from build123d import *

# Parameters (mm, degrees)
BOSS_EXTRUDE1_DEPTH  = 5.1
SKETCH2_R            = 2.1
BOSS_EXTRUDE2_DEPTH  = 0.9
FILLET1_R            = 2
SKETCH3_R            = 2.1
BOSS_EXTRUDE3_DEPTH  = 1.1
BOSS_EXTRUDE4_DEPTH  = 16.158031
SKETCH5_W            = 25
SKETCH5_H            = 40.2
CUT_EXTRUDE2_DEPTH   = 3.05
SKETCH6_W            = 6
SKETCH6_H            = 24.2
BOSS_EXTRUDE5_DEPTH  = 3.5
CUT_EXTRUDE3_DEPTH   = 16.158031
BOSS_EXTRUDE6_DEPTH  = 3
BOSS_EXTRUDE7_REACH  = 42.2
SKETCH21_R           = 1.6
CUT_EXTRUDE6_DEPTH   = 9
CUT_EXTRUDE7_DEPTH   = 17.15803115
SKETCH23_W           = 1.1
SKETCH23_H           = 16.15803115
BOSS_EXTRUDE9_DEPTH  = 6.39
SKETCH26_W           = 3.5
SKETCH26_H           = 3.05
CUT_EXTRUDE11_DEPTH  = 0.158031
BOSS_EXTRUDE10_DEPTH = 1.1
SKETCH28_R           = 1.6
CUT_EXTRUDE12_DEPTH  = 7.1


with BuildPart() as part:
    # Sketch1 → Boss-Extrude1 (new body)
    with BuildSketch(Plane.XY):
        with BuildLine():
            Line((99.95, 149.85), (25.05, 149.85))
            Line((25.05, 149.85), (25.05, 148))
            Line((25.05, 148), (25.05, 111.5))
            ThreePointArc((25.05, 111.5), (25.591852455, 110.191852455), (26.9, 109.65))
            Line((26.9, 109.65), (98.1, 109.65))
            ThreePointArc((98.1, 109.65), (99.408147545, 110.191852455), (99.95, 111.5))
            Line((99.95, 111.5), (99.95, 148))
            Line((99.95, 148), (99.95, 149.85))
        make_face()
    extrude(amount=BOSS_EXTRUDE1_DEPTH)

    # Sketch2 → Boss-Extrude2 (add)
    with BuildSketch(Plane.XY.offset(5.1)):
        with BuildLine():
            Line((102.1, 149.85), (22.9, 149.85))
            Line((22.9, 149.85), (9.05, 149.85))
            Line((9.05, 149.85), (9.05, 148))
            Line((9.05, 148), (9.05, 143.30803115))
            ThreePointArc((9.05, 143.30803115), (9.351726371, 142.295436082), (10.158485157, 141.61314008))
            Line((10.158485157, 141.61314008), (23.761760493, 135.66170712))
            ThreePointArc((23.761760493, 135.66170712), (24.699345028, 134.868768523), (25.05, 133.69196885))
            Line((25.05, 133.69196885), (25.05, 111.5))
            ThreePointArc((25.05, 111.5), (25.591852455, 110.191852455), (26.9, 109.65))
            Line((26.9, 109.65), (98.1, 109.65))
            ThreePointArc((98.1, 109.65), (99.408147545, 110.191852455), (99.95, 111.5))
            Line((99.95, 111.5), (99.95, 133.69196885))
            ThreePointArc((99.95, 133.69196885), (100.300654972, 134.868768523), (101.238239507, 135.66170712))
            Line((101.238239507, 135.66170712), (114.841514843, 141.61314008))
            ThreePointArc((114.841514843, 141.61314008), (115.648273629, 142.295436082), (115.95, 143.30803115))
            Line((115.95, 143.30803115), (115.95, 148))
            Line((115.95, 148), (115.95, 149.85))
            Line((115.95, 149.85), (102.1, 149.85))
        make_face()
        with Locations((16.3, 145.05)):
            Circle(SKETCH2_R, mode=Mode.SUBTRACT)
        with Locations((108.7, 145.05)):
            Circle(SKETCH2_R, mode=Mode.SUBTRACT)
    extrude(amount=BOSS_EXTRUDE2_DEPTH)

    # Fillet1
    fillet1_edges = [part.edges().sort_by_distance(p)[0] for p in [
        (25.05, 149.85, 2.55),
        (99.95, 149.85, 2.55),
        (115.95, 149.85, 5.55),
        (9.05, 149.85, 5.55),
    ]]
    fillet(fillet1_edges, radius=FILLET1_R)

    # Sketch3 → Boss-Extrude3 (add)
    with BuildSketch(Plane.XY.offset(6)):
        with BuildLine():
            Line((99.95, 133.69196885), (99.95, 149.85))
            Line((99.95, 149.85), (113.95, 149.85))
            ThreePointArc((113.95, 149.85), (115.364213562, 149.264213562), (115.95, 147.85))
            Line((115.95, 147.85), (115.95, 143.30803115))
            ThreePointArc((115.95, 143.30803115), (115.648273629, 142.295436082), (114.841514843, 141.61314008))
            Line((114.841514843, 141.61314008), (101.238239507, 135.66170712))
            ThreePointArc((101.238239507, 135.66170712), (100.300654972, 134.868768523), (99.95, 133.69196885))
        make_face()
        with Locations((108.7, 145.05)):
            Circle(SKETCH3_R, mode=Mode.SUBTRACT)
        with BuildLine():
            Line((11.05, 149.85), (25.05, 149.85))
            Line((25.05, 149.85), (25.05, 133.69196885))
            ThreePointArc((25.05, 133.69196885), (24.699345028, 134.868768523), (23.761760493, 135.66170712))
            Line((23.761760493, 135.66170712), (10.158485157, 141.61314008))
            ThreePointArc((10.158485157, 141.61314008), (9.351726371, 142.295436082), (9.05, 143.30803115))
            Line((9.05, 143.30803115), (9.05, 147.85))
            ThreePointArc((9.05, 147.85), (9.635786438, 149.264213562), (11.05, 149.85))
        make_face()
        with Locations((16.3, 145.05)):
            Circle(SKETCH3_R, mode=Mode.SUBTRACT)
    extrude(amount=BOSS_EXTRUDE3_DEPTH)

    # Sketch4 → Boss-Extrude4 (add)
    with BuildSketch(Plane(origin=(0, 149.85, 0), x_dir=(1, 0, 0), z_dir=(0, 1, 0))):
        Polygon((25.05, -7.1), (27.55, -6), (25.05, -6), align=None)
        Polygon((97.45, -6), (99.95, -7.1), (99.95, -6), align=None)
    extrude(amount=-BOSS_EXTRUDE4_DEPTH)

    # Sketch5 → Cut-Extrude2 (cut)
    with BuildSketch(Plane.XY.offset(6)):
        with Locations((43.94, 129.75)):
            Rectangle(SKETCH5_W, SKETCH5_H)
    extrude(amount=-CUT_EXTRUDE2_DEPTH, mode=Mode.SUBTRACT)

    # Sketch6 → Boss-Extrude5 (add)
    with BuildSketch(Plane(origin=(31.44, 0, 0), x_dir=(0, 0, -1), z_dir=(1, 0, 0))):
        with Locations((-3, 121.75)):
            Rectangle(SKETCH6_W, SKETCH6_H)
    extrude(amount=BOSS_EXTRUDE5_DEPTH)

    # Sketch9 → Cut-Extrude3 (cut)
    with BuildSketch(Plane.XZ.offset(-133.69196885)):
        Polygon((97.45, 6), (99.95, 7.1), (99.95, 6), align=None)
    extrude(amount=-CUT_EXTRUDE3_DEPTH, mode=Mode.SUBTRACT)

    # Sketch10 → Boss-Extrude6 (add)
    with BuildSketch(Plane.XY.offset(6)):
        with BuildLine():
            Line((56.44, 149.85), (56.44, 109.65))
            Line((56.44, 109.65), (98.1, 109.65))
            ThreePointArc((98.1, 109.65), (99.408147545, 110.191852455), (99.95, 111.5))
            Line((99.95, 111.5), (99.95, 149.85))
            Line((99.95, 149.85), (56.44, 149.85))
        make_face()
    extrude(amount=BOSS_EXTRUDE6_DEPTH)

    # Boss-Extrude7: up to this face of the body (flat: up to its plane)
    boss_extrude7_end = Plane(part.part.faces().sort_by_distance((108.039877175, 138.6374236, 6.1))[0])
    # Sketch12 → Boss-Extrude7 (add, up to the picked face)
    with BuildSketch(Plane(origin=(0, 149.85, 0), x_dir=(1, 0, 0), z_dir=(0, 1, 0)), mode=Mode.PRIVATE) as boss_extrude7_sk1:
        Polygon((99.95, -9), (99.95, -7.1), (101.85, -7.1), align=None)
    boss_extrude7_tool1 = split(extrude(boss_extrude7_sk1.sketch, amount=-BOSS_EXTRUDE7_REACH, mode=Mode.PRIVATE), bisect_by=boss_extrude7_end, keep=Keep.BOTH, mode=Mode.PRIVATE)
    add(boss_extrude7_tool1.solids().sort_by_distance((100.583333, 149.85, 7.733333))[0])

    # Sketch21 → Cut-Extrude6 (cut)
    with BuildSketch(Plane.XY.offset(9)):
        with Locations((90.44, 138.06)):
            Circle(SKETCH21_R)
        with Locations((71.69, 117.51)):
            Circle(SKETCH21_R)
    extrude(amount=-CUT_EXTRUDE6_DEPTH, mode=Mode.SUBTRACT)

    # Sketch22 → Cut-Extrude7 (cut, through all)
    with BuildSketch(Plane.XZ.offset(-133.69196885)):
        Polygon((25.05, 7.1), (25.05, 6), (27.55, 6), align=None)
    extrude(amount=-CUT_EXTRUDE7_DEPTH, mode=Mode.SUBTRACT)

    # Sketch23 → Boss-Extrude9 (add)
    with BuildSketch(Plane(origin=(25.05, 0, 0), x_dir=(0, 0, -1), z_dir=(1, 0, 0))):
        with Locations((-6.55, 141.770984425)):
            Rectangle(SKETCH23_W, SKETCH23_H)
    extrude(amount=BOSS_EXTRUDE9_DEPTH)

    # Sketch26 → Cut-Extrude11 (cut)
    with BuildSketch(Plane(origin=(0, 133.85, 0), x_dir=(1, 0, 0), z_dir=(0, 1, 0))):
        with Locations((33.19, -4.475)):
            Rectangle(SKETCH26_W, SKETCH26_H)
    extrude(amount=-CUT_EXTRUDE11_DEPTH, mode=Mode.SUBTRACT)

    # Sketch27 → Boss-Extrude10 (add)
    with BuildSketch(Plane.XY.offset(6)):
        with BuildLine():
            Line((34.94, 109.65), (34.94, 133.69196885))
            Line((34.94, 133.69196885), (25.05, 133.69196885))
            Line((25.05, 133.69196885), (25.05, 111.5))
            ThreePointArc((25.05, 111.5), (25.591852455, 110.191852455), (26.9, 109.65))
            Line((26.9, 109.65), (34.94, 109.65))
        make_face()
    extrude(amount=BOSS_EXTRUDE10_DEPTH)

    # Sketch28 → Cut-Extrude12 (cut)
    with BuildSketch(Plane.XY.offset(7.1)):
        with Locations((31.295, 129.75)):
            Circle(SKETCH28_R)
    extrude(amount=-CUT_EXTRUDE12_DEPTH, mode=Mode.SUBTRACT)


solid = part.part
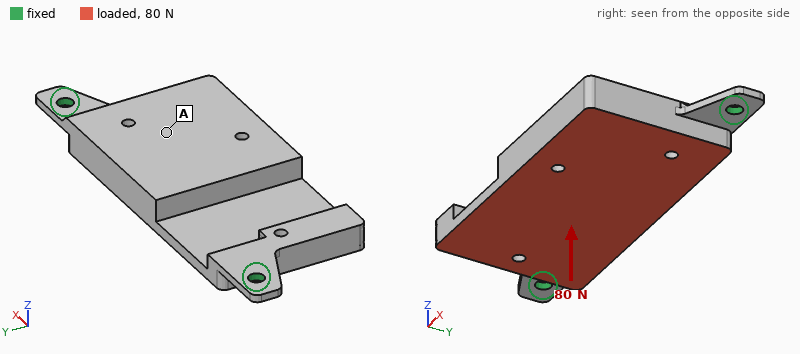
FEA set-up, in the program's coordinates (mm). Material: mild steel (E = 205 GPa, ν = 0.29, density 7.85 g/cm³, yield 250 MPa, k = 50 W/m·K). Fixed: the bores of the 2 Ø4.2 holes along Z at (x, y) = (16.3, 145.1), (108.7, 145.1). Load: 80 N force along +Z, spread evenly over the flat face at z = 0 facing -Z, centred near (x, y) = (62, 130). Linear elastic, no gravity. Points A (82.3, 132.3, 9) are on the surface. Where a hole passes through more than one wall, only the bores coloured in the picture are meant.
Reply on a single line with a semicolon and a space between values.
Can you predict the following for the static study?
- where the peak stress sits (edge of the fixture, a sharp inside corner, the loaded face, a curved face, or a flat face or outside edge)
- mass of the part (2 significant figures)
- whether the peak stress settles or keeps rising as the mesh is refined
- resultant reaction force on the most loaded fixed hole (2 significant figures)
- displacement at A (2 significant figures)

edge of the fixture; 170 g; keeps rising; 120 N; 19 µm
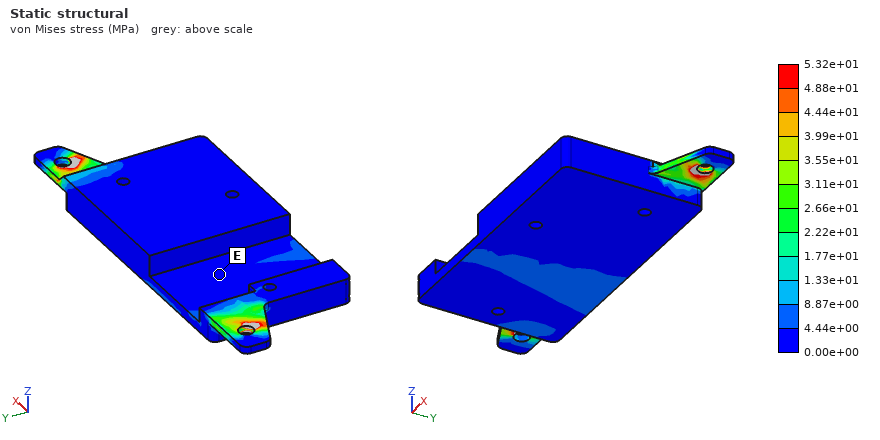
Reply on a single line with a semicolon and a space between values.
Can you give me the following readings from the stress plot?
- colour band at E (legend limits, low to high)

0.00e+00 to 4.44e+00 MPa
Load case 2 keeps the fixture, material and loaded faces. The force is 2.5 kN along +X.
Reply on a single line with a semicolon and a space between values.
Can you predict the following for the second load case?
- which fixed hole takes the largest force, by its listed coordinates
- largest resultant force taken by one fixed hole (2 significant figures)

(108.7, 145.1); 1.7 kN
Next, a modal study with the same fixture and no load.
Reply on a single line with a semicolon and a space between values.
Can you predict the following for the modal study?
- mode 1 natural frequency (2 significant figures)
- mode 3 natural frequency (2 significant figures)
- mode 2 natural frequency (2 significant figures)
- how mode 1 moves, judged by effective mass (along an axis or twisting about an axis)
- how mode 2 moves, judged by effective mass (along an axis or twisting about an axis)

610 Hz; 3200 Hz; 2400 Hz; along Z; along Z
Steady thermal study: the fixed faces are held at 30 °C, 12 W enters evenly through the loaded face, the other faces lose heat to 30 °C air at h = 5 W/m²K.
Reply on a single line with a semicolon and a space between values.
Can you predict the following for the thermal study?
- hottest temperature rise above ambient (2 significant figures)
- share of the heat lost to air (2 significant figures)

55 K; 11 %
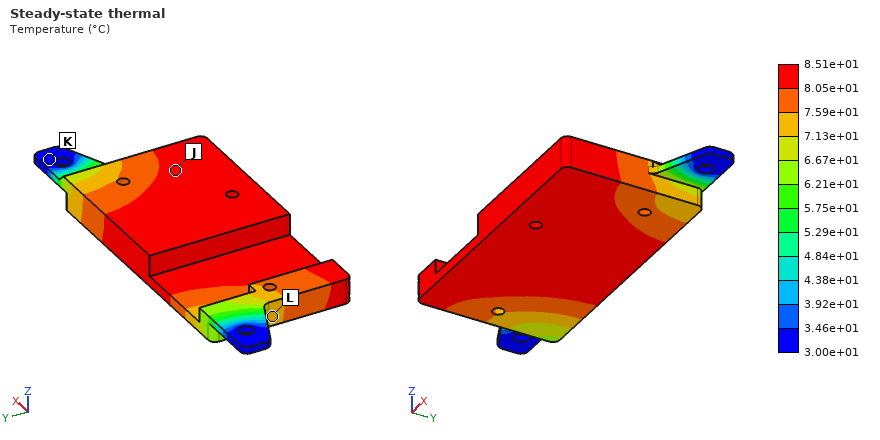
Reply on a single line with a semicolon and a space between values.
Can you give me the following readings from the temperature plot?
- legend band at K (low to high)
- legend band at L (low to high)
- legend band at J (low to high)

3.00e+01 to 3.46e+01 °C; 7.13e+01 to 7.59e+01 °C; 8.05e+01 to 8.51e+01 °C
